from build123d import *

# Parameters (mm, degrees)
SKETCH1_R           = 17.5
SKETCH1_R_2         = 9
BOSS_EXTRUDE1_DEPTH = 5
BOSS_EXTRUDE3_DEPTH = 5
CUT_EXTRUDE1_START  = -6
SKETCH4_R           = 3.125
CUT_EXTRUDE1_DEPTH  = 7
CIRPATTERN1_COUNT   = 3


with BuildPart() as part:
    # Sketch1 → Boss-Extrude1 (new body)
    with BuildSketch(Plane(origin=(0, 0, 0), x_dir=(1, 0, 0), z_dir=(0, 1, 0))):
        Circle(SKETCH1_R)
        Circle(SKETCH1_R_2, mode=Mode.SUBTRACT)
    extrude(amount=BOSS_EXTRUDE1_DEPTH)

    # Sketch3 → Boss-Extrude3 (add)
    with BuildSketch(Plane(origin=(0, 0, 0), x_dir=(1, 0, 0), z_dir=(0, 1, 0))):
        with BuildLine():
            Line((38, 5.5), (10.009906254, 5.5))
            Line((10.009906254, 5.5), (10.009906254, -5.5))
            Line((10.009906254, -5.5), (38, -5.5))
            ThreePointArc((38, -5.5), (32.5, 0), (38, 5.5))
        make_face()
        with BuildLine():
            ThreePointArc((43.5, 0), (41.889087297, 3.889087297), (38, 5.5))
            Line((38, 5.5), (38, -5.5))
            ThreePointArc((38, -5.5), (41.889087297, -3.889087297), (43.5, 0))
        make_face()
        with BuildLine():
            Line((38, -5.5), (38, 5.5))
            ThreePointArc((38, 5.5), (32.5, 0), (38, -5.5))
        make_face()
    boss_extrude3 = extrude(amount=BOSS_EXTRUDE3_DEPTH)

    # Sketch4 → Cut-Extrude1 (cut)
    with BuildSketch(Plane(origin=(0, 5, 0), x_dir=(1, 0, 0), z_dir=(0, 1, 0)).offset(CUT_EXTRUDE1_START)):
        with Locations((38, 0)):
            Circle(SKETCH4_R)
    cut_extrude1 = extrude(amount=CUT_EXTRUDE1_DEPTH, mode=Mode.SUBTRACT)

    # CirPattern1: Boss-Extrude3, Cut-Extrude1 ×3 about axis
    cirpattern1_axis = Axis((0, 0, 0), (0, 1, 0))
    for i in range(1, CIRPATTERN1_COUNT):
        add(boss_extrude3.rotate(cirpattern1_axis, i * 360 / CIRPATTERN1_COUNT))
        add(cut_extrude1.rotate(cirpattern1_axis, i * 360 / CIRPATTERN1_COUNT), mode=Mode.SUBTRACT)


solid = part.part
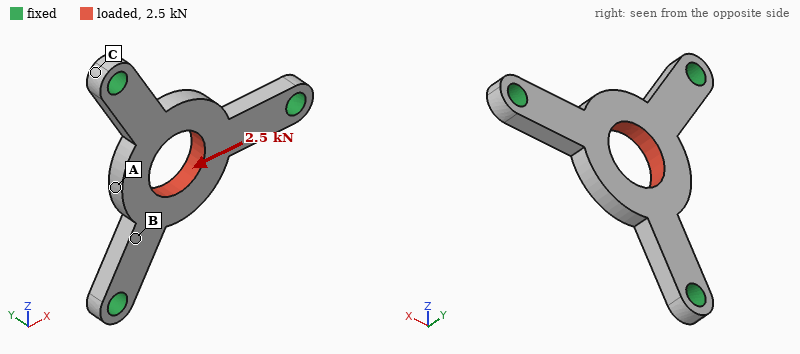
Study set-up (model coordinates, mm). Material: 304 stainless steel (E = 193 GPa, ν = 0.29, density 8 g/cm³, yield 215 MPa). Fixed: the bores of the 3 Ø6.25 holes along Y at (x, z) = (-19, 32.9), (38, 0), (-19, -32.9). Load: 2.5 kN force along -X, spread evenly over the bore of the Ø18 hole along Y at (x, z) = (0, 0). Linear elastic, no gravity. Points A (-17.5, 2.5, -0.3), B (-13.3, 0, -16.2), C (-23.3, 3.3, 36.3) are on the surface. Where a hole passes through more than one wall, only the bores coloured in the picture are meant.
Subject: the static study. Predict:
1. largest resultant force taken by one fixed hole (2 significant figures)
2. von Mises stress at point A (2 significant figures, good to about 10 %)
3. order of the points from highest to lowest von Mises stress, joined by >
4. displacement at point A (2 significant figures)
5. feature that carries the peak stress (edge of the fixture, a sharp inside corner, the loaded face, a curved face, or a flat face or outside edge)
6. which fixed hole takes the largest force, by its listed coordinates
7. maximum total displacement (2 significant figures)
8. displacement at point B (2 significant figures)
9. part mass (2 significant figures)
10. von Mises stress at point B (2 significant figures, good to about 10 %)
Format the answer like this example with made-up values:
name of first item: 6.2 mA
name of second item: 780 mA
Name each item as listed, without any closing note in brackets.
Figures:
largest resultant force taken by one fixed hole: 1.4 kN
von Mises stress at point A: 31 MPa
order of the points from highest to lowest von Mises stress, joined by >: A > B > C
displacement at point A: 10 µm
feature that carries the peak stress: the loaded face
which fixed hole takes the largest force, by its listed coordinates: (38, 0)
maximum total displacement: 11 µm
displacement at point B: 5.1 µm
part mass: 58 g
von Mises stress at point B: 15 MPa
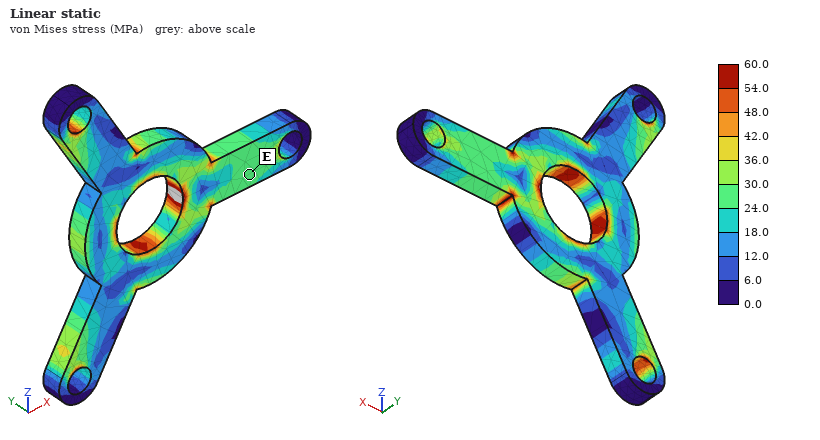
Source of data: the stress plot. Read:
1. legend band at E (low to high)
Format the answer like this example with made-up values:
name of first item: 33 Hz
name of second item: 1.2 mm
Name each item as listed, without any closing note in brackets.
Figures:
legend band at E: 24.0 to 30.0 MPa
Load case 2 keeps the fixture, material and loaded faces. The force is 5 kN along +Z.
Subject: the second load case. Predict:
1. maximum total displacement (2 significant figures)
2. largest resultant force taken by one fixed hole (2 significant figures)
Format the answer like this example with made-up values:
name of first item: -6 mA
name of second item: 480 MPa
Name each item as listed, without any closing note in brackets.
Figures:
maximum total displacement: 20 µm
largest resultant force taken by one fixed hole: 2.5 kN
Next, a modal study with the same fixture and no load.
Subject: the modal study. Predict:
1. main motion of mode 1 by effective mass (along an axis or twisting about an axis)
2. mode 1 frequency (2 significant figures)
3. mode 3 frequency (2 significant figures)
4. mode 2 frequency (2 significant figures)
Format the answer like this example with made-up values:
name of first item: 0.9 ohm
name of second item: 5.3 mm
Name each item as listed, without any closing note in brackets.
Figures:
main motion of mode 1 by effective mass: along Y
mode 1 frequency: 5100 Hz
mode 3 frequency: 9200 Hz
mode 2 frequency: 9200 Hz
